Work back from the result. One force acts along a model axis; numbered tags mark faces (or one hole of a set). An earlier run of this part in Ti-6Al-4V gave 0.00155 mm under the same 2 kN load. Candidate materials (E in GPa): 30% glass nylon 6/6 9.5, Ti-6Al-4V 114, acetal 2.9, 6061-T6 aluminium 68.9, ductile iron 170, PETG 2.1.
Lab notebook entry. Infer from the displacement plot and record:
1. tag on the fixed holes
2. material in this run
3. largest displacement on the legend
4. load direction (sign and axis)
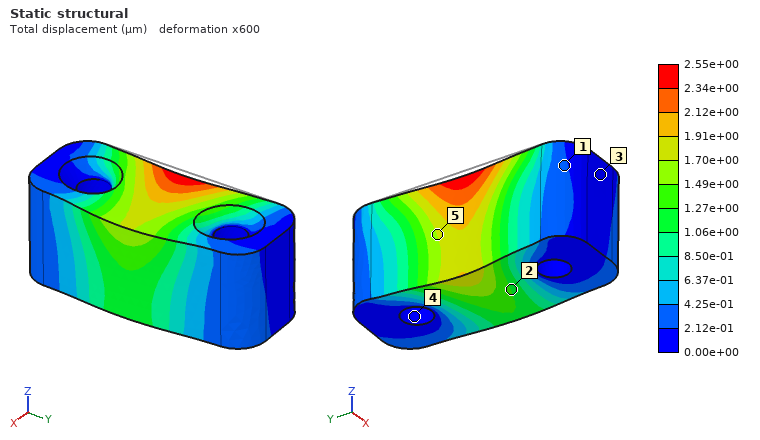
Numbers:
4
6061-T6 aluminium
2.55e+00 µm
+X
